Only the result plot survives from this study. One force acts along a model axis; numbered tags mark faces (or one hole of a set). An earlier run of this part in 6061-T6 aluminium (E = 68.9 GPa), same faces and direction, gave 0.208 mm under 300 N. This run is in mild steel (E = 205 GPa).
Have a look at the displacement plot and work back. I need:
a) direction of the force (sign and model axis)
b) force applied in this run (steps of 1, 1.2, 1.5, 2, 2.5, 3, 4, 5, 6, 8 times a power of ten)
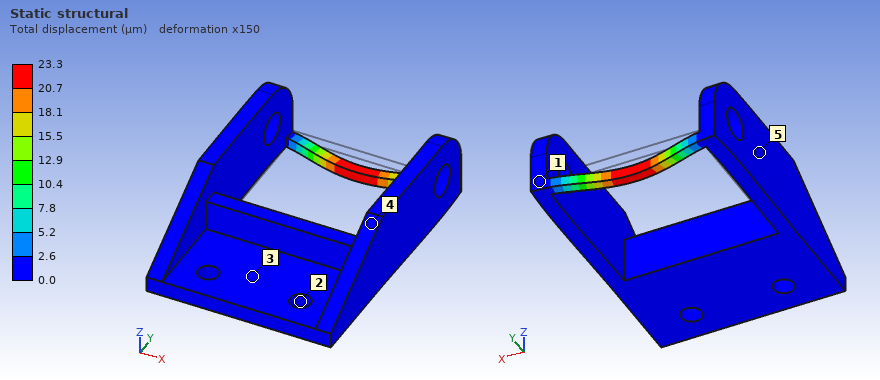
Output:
-Y
100 N
